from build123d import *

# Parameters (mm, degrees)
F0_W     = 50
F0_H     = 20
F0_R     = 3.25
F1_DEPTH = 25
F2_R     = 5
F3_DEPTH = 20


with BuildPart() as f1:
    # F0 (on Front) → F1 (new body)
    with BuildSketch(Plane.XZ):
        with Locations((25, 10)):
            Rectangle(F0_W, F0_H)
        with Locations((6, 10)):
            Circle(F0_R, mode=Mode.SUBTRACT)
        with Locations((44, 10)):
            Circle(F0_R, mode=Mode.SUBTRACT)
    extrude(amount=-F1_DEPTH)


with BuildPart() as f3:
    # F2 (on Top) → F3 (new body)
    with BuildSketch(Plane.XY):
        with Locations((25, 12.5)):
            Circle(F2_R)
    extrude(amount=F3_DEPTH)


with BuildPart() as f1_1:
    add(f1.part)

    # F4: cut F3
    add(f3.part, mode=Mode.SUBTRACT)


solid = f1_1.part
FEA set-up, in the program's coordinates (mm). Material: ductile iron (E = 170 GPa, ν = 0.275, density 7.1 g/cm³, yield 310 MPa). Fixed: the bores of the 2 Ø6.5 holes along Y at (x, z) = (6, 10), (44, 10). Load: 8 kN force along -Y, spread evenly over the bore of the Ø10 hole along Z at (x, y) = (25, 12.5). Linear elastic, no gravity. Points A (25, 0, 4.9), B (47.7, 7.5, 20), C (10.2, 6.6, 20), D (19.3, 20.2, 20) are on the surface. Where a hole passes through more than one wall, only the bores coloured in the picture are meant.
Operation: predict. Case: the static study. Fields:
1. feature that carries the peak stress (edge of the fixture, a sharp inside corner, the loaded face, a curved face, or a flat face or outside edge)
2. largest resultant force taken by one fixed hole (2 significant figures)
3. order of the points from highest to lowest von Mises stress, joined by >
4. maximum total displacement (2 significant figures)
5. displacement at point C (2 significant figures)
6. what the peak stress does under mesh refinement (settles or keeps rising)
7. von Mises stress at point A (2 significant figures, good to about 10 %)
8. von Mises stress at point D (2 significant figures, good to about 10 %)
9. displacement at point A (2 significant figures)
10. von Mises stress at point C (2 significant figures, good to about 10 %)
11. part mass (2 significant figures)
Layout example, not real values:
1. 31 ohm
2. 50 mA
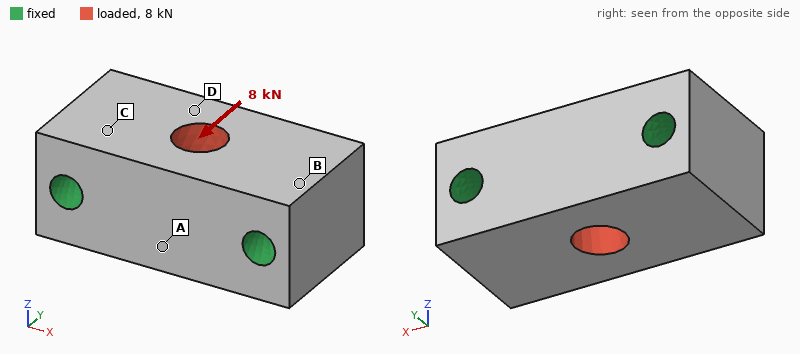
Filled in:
1. edge of the fixture
2. 4.0 kN
3. A > D > C > B
4. 2.9 µm
5. 0.69 µm
6. keeps rising
7. 21 MPa
8. 14 MPa
9. 2.5 µm
10. 9.3 MPa
11. 150 g
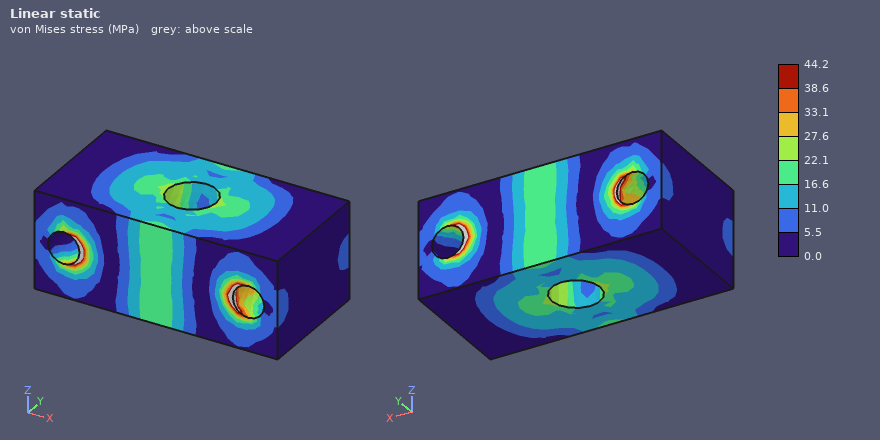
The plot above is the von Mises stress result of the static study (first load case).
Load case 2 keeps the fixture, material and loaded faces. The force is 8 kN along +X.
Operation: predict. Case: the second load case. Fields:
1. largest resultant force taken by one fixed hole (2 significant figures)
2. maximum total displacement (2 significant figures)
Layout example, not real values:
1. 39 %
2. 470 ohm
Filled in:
1. 4.0 kN
2. 1.1 µm
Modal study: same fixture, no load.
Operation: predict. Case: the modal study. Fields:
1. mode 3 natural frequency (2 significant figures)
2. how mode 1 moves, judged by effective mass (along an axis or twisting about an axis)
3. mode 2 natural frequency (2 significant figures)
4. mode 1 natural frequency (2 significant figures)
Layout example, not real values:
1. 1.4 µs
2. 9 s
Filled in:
1. 39 kHz
2. along Z
3. 39 kHz
4. 31 kHz
